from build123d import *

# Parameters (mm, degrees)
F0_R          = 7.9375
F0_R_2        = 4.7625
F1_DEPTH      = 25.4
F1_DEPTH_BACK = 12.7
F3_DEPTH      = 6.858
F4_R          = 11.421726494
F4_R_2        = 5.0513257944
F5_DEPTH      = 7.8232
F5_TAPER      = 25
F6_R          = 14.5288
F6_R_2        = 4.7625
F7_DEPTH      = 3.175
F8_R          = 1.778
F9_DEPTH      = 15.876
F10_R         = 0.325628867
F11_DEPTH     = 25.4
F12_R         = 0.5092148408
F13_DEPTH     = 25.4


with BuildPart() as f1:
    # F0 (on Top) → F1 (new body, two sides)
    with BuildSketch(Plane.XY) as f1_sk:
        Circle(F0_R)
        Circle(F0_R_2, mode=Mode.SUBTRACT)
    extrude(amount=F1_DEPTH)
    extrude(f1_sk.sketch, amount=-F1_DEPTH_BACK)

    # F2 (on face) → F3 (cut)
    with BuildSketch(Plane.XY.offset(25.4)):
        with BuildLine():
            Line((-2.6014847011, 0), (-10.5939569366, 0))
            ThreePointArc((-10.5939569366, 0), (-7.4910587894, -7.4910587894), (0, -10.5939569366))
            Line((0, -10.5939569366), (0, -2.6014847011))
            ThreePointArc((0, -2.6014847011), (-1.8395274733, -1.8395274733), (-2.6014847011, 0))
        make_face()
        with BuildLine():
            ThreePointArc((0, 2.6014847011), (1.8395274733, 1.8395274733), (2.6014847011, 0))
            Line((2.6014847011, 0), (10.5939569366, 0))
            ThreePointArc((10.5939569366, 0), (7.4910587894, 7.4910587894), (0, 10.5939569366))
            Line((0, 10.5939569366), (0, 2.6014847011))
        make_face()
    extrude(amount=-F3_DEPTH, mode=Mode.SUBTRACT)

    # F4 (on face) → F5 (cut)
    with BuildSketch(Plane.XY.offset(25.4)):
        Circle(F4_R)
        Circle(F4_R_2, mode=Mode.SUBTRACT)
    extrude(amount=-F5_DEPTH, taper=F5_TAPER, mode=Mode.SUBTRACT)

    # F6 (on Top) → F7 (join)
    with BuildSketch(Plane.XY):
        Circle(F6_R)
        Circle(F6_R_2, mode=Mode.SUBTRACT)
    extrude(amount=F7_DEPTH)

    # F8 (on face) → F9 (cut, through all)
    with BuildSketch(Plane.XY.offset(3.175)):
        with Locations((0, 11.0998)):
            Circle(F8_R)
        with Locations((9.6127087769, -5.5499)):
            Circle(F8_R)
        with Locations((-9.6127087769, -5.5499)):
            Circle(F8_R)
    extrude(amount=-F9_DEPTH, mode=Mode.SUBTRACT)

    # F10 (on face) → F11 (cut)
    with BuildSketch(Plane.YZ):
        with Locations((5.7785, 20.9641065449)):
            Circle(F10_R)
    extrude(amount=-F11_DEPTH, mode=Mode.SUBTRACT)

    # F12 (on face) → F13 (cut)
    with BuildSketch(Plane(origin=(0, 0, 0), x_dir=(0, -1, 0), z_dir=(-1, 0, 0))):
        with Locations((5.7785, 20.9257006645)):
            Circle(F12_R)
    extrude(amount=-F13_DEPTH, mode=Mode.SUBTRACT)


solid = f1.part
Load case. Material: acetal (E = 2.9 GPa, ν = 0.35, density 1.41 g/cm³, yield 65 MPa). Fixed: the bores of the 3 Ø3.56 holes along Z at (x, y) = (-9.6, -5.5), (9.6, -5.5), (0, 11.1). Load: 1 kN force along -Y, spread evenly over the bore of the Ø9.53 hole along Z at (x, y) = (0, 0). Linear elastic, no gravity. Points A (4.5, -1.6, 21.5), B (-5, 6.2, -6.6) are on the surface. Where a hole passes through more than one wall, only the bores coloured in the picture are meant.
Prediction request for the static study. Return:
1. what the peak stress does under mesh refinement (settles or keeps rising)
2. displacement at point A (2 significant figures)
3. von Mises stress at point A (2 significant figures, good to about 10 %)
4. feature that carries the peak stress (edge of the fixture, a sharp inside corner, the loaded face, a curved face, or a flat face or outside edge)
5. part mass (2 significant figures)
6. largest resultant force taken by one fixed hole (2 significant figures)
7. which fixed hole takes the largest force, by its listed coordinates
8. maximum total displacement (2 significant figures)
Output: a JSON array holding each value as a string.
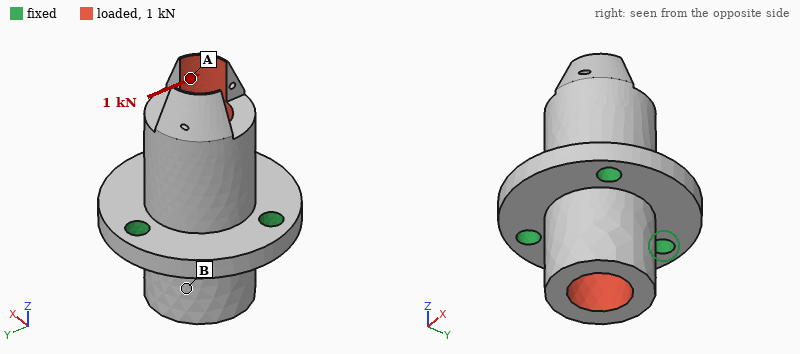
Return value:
["keeps rising", "0.26 mm", "10 MPa", "edge of the fixture", "7.9 g", "400 N", "(0, 11.1)", "0.38 mm"]
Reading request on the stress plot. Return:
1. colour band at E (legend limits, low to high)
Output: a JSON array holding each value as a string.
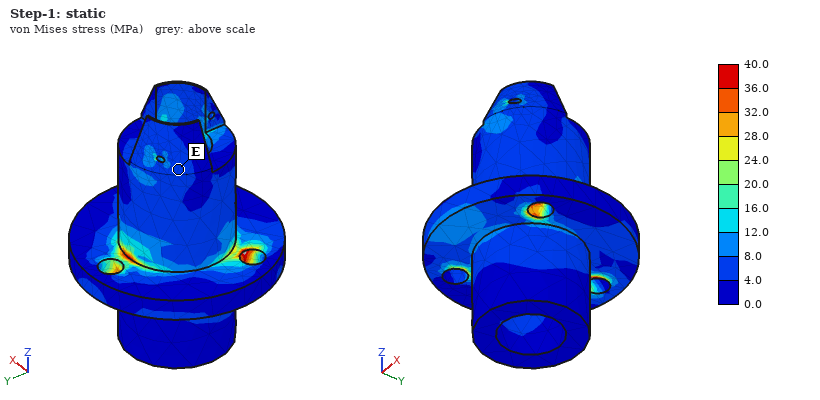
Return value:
["4.0 to 8.0 MPa"]
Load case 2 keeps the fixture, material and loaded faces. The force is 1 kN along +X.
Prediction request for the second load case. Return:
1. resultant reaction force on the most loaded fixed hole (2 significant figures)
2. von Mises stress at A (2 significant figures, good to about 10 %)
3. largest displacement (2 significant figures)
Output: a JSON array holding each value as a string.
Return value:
["380 N", "6.3 MPa", "0.38 mm"]
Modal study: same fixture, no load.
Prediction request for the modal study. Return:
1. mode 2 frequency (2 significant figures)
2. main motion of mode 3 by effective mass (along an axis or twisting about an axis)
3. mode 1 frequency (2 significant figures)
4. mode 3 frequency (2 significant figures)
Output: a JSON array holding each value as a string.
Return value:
["4400 Hz", "along Z", "4400 Hz", "7900 Hz"]
